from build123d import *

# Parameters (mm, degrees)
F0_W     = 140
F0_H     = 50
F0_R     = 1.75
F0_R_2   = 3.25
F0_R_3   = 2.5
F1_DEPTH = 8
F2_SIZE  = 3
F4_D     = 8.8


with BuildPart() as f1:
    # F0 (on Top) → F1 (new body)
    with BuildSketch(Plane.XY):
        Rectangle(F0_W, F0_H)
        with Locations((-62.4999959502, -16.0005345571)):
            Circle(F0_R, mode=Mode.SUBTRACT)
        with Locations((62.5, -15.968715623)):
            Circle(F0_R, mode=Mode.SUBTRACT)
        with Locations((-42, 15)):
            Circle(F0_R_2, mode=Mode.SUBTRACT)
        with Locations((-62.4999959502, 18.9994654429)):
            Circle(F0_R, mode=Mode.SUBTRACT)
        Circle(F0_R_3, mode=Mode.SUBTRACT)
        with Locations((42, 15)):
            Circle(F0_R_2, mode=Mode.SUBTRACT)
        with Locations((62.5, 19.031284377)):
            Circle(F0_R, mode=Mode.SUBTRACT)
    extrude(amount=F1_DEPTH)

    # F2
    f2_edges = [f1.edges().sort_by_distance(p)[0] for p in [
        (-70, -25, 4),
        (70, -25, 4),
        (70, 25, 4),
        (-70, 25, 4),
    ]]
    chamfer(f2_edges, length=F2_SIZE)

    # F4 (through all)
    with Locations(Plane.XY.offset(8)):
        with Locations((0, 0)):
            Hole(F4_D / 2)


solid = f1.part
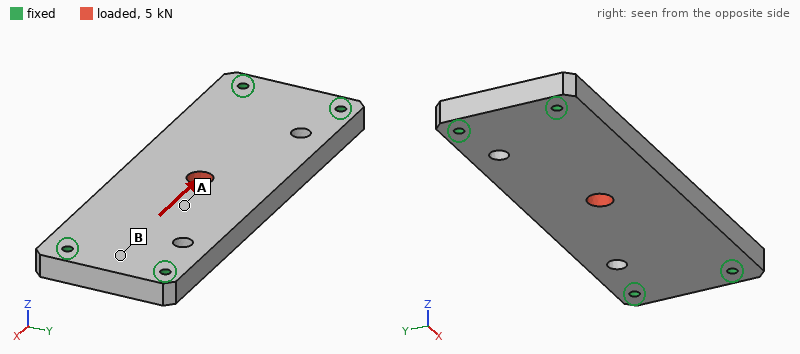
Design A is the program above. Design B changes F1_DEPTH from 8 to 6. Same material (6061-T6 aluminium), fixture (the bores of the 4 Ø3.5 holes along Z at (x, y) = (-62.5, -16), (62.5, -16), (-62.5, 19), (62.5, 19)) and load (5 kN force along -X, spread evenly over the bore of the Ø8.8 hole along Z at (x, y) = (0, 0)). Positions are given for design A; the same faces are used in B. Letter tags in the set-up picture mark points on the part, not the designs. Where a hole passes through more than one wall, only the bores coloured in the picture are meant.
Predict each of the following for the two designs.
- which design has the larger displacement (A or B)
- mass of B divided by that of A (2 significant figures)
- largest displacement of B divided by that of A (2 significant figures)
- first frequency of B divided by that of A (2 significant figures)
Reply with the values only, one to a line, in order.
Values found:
B
0.75
1.3
0.78
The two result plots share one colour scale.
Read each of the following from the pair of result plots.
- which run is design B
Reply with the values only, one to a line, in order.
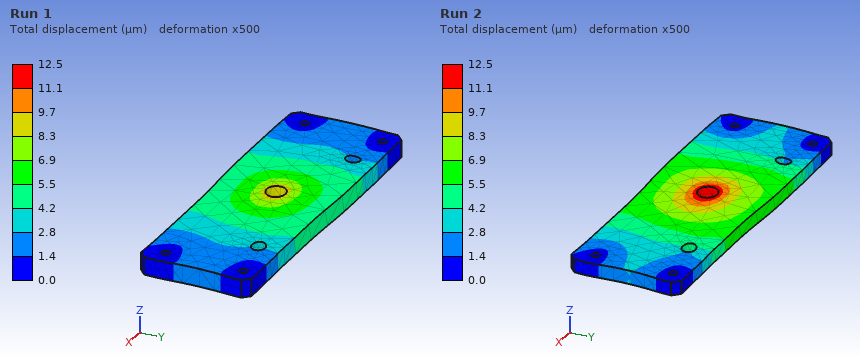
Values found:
Run 2
